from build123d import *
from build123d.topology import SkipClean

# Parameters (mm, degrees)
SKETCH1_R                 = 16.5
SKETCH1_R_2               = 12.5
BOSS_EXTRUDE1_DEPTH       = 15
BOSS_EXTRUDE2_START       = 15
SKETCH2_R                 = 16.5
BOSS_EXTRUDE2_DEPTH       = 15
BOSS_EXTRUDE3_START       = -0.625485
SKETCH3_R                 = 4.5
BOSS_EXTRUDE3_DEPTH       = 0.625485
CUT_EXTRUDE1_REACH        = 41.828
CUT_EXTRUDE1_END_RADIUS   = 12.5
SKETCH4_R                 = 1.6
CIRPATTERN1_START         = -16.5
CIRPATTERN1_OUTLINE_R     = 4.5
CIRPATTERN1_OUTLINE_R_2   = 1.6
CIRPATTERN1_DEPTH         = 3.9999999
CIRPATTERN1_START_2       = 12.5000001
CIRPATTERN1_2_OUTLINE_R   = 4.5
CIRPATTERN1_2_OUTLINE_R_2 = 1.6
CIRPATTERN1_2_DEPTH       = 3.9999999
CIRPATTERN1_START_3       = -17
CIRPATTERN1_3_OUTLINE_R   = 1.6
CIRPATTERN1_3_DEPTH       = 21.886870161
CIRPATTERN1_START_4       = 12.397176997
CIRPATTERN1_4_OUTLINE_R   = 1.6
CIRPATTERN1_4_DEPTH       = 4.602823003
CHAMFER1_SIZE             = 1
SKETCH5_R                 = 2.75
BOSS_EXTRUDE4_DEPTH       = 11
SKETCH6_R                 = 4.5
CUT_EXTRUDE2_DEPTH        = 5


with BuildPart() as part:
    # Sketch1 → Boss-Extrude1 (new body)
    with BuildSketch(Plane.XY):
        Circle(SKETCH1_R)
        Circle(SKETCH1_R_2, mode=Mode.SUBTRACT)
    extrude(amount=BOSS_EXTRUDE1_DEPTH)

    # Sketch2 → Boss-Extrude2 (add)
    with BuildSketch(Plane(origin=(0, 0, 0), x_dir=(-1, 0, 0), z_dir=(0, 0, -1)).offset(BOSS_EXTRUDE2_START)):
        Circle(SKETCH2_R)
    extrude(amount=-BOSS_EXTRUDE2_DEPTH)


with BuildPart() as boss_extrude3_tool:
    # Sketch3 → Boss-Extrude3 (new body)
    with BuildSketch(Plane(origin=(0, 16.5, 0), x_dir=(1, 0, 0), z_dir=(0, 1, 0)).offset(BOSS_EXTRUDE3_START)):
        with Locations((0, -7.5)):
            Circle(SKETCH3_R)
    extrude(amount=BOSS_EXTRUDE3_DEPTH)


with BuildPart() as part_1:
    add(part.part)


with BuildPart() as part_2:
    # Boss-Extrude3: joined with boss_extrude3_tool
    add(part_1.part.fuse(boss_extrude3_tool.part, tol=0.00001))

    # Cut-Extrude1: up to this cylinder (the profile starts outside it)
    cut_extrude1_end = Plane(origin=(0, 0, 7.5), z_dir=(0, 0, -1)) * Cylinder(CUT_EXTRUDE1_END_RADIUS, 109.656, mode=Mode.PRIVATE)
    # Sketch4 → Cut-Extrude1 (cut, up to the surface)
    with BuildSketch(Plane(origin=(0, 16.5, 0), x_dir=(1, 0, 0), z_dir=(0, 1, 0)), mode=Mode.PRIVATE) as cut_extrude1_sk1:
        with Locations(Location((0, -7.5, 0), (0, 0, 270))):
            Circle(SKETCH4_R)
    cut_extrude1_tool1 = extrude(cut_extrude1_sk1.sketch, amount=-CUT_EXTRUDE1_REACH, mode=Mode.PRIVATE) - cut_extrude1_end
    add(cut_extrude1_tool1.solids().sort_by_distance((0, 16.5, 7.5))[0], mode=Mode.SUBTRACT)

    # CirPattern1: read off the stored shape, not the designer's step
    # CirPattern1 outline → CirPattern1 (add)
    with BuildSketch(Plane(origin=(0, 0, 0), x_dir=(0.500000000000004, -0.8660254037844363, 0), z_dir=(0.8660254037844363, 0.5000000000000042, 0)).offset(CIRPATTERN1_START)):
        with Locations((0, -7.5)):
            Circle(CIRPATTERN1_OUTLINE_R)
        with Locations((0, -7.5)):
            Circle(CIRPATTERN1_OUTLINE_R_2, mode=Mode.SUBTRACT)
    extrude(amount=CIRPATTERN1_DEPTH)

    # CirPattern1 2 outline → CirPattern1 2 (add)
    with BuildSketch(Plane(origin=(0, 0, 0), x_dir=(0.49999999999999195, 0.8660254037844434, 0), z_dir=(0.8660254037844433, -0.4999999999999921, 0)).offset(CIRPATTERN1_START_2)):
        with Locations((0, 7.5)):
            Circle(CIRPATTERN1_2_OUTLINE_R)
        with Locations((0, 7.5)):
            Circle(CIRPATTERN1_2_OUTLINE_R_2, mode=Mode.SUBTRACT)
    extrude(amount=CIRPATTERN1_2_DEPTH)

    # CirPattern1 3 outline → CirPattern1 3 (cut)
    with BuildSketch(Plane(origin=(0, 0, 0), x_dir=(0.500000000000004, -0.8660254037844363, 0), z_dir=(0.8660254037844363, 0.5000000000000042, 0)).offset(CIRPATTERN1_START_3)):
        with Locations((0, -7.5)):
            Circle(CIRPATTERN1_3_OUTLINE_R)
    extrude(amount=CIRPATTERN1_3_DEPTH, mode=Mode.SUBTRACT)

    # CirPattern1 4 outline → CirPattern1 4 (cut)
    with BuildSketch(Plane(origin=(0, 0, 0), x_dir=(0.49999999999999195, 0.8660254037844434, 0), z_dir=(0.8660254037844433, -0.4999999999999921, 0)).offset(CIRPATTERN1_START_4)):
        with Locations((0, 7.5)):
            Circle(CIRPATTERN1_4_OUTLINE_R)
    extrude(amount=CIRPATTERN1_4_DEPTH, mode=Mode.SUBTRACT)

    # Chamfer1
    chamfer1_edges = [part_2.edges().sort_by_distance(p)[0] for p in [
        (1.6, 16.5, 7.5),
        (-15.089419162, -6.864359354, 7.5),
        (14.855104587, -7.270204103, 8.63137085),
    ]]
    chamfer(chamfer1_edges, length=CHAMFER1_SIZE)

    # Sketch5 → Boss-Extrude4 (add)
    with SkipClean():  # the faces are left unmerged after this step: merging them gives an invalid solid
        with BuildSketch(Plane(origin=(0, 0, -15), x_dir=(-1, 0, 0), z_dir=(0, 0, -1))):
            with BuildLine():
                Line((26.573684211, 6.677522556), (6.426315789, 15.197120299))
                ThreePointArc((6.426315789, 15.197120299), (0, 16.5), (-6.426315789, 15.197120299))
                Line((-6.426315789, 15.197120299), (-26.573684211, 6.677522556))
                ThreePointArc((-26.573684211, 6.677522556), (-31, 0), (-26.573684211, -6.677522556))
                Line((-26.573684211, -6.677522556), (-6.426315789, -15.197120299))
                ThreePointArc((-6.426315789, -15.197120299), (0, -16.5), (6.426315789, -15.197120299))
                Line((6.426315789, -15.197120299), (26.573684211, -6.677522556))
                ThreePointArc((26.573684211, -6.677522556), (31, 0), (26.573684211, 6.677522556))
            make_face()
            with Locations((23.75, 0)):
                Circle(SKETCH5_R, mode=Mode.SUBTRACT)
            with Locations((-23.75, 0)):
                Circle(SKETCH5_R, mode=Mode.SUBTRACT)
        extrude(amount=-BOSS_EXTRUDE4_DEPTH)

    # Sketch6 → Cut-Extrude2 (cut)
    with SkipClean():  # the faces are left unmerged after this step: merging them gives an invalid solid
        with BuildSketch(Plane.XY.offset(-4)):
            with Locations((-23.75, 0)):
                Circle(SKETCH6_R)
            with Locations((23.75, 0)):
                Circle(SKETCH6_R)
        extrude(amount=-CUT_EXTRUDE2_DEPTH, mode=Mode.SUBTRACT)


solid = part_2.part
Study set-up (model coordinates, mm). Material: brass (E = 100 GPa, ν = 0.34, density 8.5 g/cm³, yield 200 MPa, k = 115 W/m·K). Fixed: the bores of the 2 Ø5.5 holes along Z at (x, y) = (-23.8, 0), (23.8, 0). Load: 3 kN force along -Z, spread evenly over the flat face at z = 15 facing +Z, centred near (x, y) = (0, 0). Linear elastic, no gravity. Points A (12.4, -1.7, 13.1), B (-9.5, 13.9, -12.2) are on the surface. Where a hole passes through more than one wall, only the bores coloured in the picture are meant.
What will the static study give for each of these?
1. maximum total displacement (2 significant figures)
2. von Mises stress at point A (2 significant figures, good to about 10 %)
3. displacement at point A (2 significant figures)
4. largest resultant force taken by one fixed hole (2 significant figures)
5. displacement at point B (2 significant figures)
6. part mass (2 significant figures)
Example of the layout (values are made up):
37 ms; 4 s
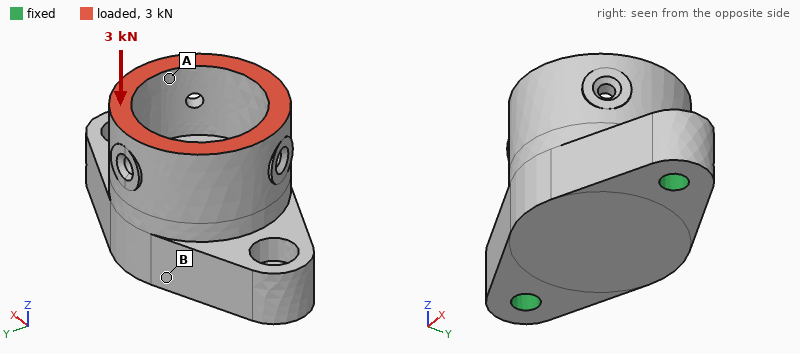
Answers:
9.5 µm; 18 MPa; 7.1 µm; 1.8 kN; 6.1 µm; 200 g
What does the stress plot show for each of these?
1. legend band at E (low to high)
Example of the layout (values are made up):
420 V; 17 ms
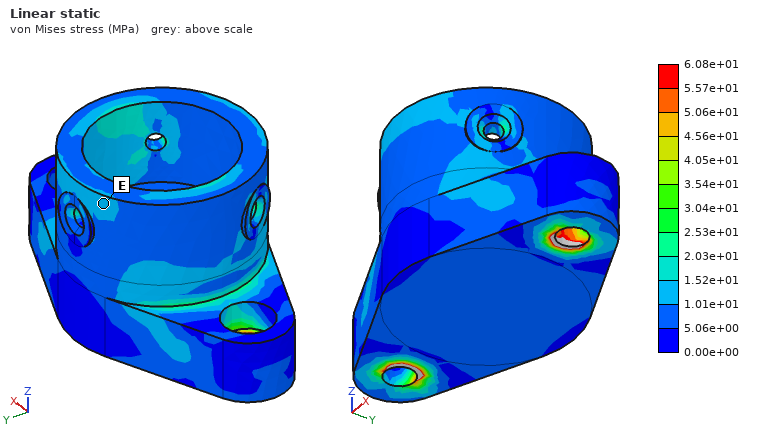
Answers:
1.01e+01 to 1.52e+01 MPa
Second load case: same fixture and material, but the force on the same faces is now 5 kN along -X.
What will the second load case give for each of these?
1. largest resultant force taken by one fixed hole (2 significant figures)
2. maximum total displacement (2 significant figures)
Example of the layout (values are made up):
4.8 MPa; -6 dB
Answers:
4.0 kN; 39 µm
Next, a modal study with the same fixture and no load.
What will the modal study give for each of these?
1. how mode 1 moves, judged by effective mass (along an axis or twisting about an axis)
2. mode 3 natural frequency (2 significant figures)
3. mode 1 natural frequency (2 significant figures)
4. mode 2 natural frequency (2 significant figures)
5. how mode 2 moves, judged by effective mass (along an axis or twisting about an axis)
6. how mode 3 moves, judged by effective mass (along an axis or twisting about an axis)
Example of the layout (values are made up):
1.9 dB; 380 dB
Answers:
along Y; 12 kHz; 3700 Hz; 8600 Hz; along Z; along X
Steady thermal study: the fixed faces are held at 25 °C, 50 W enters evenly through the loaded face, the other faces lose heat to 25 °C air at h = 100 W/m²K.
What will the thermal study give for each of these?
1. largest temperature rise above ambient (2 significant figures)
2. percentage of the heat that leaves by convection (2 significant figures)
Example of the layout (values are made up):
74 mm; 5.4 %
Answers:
34 K; 23 %
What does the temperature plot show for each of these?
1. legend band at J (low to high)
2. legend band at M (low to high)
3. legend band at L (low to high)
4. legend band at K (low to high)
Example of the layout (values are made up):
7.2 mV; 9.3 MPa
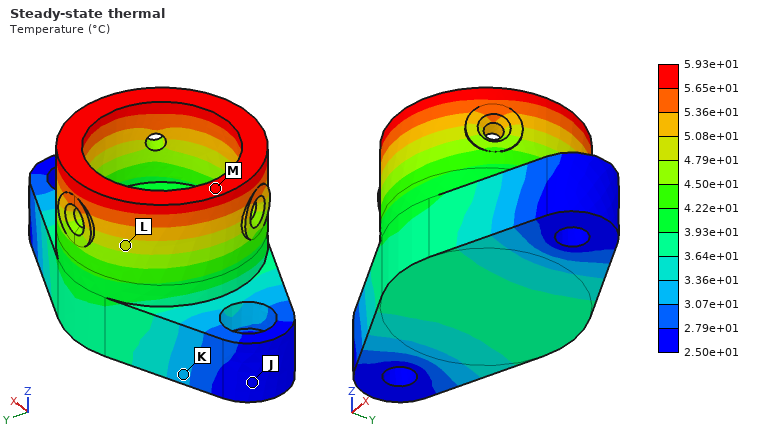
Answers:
2.50e+01 to 2.79e+01 °C; 5.65e+01 to 5.93e+01 °C; 4.79e+01 to 5.08e+01 °C; 3.07e+01 to 3.36e+01 °C
